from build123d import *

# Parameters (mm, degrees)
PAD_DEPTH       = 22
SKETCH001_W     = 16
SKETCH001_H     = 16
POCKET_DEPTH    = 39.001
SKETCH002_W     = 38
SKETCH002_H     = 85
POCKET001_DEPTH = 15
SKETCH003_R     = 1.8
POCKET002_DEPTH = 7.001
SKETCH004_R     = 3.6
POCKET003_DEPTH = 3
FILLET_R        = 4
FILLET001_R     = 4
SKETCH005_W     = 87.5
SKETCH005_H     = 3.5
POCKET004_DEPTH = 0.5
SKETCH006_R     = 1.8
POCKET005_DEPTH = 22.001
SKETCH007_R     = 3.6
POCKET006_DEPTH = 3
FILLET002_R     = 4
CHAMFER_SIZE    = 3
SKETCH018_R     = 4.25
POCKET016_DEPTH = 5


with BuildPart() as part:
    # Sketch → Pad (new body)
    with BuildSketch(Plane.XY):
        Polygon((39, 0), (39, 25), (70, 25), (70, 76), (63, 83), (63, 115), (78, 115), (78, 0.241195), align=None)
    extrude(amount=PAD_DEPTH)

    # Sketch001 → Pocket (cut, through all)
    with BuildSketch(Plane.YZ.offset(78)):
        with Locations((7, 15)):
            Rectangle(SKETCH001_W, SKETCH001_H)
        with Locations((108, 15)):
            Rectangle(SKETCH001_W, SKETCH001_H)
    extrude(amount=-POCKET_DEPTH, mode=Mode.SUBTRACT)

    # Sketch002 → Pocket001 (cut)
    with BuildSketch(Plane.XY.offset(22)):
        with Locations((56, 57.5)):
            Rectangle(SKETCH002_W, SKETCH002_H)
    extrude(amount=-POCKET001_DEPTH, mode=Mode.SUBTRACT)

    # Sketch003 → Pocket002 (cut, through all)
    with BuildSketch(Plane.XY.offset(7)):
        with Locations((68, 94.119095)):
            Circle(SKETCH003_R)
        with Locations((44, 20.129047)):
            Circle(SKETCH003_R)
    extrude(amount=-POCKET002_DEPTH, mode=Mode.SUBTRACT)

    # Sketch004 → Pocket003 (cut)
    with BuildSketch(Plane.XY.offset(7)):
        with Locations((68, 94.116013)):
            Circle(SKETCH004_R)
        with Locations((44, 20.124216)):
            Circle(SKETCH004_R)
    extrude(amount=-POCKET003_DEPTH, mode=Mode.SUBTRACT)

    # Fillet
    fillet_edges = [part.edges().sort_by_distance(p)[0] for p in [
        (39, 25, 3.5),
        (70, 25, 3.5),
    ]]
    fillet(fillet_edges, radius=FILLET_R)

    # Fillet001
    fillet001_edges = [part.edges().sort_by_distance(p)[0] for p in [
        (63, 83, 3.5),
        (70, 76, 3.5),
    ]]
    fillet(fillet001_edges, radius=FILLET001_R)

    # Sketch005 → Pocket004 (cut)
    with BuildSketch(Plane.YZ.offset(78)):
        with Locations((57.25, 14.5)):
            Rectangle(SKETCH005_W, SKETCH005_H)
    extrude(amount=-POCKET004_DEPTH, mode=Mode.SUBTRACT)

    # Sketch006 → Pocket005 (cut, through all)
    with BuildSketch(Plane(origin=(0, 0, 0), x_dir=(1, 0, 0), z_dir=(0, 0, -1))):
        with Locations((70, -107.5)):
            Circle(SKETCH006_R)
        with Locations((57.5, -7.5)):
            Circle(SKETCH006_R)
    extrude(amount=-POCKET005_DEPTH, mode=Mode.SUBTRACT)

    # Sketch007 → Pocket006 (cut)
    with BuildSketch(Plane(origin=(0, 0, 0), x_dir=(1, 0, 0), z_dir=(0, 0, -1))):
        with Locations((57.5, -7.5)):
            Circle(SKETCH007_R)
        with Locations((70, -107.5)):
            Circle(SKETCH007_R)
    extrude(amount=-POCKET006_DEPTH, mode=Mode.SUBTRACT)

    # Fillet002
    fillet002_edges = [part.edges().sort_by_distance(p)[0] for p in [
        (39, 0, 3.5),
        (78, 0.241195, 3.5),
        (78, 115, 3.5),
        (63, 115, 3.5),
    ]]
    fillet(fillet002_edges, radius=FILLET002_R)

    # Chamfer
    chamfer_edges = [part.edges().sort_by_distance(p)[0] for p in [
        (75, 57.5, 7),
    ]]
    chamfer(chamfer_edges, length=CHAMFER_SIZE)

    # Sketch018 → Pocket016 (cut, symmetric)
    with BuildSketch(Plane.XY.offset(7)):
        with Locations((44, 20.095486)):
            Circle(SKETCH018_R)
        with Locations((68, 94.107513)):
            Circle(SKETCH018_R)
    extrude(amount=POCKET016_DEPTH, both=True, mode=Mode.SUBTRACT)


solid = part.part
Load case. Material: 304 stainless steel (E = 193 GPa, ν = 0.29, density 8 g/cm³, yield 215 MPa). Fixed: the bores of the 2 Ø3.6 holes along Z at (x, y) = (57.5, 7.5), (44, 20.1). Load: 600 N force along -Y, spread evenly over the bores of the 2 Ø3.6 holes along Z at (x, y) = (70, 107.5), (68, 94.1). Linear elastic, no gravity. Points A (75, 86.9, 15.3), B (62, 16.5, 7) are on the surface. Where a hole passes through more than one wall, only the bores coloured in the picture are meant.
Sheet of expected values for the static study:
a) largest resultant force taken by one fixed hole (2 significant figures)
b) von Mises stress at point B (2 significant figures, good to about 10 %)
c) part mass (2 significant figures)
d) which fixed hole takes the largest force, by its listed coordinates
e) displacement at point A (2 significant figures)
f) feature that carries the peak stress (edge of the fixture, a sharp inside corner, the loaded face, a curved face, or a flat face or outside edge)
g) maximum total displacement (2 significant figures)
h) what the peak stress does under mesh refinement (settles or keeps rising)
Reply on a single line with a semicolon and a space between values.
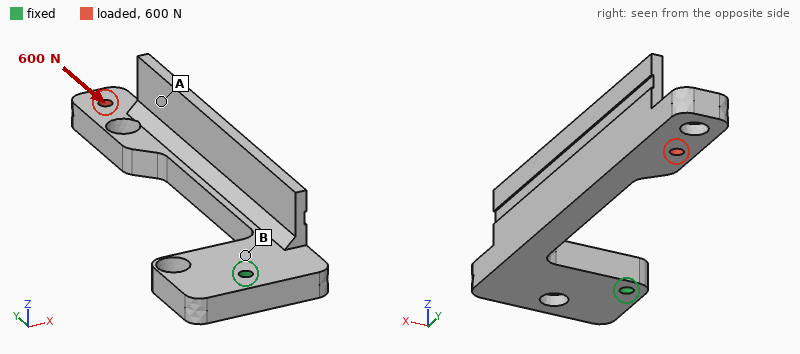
780 N; 9.3 MPa; 130 g; (57.5, 7.5); 0.070 mm; edge of the fixture; 0.14 mm; keeps rising
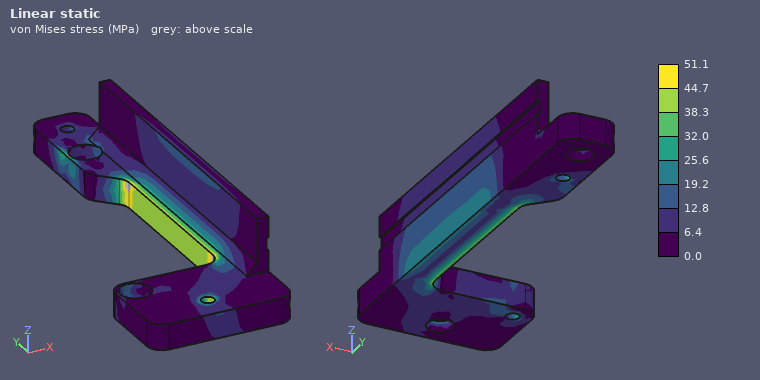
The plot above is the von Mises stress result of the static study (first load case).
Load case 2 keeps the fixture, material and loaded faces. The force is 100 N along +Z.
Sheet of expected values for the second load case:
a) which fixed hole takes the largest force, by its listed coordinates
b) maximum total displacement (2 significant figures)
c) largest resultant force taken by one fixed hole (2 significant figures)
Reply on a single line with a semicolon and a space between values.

(44, 20.1); 0.26 mm; 240 N
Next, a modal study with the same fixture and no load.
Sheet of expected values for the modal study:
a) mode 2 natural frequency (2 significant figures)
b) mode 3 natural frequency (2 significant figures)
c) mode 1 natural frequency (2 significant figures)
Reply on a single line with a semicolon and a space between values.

630 Hz; 2400 Hz; 500 Hz
